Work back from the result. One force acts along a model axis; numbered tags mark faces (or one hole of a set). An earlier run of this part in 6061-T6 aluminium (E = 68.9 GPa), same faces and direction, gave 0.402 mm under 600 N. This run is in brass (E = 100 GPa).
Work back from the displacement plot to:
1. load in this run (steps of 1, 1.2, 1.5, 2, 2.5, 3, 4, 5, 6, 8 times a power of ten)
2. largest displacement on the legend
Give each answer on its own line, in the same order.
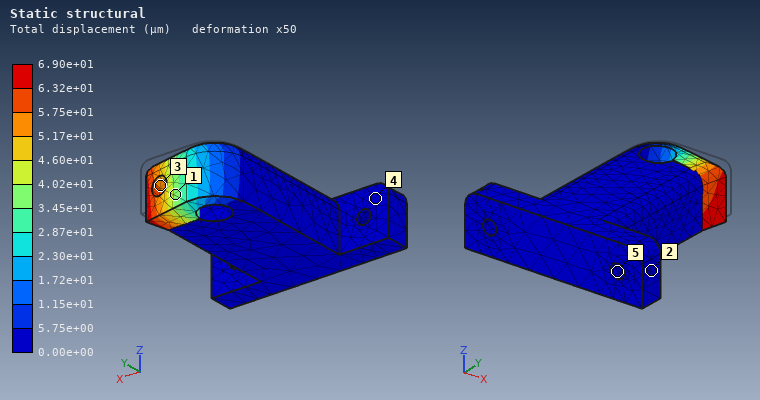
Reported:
150 N
6.90e+01 µm
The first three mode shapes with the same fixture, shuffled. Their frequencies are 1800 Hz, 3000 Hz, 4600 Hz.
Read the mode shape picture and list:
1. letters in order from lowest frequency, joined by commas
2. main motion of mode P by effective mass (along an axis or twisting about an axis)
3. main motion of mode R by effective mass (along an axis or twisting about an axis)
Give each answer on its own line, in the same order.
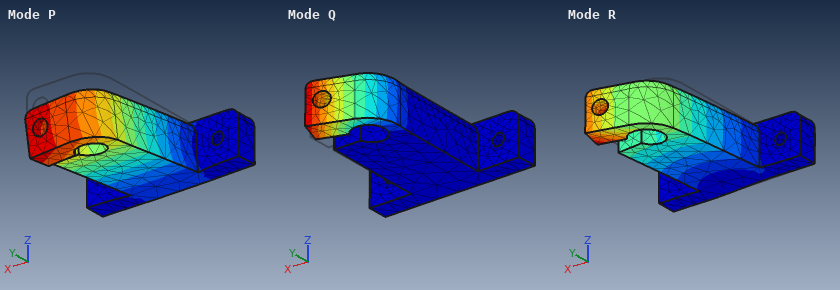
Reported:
P, Q, R
along Z
along X
